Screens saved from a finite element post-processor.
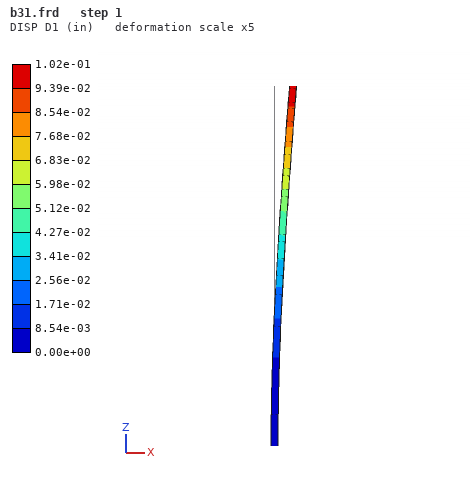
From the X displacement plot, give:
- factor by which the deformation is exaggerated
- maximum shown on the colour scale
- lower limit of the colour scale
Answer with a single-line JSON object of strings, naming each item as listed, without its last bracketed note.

{"factor by which the deformation is exaggerated": "5", "maximum shown on the colour scale": "1.02e-01 in", "lower limit of the colour scale": "0.00e+00 in"}
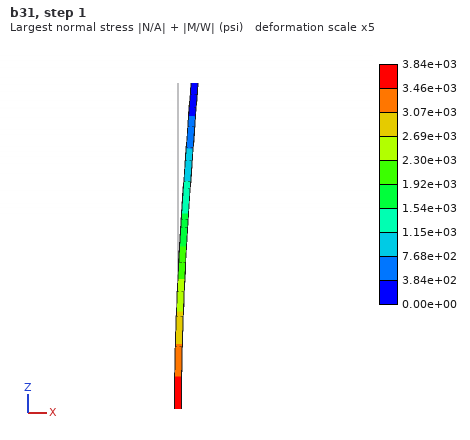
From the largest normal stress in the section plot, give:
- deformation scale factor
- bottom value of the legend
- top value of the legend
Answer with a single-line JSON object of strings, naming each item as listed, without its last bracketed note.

{"deformation scale factor": "5", "bottom value of the legend": "0.00e+00 psi", "top value of the legend": "3.84e+03 psi"}
